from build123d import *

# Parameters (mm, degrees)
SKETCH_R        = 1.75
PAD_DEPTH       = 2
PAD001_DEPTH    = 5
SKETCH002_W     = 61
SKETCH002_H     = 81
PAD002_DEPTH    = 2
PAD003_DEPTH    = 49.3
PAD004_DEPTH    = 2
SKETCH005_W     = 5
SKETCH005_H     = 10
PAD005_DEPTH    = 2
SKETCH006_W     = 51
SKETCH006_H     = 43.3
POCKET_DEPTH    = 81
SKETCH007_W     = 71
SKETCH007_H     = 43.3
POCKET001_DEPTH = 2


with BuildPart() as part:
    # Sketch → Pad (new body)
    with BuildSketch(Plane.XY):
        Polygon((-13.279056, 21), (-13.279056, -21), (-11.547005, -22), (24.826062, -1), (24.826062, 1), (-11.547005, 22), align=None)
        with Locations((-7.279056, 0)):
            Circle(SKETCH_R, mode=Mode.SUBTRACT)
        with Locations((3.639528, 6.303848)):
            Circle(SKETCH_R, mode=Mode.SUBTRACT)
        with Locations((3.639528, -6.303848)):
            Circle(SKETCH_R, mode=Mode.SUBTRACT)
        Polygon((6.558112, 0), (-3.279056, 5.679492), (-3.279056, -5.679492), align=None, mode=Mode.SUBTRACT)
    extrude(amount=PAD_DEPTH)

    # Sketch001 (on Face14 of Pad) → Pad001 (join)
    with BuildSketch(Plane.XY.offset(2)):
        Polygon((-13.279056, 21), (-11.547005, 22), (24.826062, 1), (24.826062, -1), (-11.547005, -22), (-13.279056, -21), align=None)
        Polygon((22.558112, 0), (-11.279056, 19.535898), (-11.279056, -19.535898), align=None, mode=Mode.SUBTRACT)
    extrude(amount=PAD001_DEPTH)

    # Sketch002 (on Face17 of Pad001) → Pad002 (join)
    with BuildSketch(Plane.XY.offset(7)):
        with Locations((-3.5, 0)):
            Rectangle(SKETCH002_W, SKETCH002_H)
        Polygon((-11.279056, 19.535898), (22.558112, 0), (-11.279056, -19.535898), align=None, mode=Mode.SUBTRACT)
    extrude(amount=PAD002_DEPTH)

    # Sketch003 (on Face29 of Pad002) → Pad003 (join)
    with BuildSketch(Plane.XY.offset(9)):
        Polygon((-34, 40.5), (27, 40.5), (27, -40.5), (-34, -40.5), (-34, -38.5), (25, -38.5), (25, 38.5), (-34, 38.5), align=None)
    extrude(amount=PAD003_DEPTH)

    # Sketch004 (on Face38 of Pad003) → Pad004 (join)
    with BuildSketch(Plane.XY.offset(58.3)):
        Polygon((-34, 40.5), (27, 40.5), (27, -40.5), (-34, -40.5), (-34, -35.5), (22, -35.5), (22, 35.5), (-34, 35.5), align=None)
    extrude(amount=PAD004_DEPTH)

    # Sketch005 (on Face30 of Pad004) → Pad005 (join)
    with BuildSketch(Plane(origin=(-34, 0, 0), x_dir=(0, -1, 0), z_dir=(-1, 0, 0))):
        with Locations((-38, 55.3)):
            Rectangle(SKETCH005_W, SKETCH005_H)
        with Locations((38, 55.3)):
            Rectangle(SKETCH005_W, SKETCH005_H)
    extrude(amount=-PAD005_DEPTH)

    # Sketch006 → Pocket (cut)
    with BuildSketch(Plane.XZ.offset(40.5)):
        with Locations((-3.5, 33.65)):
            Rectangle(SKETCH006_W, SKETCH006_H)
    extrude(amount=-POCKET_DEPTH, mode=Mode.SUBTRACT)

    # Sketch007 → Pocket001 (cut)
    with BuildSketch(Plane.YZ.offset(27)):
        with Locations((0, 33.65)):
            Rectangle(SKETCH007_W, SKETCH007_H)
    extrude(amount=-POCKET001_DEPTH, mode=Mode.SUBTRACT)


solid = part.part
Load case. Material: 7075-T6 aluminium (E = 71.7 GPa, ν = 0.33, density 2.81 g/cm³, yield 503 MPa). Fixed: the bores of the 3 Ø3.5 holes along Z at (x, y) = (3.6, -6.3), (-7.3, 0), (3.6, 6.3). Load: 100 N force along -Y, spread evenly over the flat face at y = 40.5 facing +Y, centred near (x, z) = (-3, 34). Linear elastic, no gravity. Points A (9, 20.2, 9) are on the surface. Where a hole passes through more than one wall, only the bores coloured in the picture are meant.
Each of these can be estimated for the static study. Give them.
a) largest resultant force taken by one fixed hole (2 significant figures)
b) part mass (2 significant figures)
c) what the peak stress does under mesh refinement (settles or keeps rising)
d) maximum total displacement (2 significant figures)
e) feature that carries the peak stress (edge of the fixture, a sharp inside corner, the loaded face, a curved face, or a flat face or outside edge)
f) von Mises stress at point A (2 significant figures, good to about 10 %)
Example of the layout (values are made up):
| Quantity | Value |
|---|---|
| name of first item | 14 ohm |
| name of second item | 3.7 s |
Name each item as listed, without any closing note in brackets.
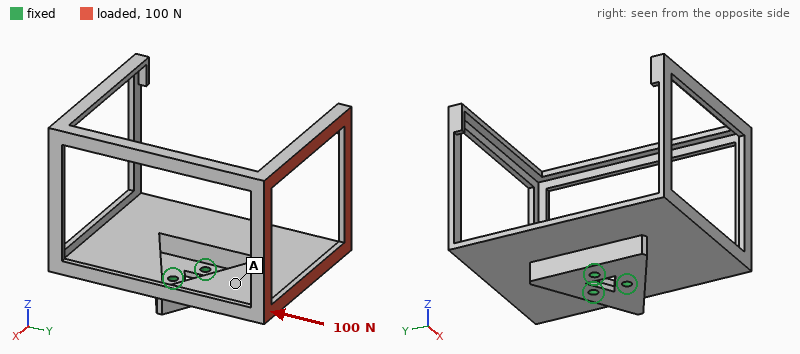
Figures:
| Quantity | Value |
|---|---|
| largest resultant force taken by one fixed hole | 180 N |
| part mass | 51 g |
| what the peak stress does under mesh refinement | keeps rising |
| maximum total displacement | 1.3 mm |
| feature that carries the peak stress | a sharp inside corner |
| von Mises stress at point A | 17 MPa |
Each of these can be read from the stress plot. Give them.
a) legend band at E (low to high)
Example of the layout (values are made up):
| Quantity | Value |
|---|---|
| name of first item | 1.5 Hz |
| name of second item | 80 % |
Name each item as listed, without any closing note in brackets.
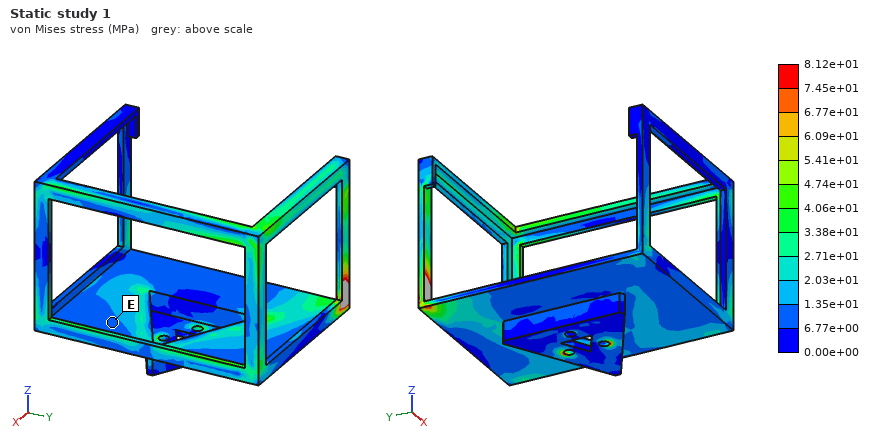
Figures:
| Quantity | Value |
|---|---|
| legend band at E | 6.77e+00 to 1.35e+01 MPa |
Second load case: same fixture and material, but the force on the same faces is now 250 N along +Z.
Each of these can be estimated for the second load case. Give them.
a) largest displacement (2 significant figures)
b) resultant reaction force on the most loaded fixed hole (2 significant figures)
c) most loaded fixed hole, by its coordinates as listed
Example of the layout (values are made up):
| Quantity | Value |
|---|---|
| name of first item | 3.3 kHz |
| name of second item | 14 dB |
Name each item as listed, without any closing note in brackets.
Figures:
| Quantity | Value |
|---|---|
| largest displacement | 1.0 mm |
| resultant reaction force on the most loaded fixed hole | 590 N |
| most loaded fixed hole, by its coordinates as listed | (3.6, 6.3) |
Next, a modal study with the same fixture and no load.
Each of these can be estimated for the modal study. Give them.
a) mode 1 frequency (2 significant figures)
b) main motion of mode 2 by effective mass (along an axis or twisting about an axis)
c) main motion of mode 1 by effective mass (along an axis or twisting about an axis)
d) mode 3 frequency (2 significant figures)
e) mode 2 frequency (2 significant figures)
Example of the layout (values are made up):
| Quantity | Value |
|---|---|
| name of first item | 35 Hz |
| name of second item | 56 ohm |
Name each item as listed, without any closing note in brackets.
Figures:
| Quantity | Value |
|---|---|
| mode 1 frequency | 410 Hz |
| main motion of mode 2 by effective mass | along X |
| main motion of mode 1 by effective mass | along Y |
| mode 3 frequency | 730 Hz |
| mode 2 frequency | 540 Hz |
